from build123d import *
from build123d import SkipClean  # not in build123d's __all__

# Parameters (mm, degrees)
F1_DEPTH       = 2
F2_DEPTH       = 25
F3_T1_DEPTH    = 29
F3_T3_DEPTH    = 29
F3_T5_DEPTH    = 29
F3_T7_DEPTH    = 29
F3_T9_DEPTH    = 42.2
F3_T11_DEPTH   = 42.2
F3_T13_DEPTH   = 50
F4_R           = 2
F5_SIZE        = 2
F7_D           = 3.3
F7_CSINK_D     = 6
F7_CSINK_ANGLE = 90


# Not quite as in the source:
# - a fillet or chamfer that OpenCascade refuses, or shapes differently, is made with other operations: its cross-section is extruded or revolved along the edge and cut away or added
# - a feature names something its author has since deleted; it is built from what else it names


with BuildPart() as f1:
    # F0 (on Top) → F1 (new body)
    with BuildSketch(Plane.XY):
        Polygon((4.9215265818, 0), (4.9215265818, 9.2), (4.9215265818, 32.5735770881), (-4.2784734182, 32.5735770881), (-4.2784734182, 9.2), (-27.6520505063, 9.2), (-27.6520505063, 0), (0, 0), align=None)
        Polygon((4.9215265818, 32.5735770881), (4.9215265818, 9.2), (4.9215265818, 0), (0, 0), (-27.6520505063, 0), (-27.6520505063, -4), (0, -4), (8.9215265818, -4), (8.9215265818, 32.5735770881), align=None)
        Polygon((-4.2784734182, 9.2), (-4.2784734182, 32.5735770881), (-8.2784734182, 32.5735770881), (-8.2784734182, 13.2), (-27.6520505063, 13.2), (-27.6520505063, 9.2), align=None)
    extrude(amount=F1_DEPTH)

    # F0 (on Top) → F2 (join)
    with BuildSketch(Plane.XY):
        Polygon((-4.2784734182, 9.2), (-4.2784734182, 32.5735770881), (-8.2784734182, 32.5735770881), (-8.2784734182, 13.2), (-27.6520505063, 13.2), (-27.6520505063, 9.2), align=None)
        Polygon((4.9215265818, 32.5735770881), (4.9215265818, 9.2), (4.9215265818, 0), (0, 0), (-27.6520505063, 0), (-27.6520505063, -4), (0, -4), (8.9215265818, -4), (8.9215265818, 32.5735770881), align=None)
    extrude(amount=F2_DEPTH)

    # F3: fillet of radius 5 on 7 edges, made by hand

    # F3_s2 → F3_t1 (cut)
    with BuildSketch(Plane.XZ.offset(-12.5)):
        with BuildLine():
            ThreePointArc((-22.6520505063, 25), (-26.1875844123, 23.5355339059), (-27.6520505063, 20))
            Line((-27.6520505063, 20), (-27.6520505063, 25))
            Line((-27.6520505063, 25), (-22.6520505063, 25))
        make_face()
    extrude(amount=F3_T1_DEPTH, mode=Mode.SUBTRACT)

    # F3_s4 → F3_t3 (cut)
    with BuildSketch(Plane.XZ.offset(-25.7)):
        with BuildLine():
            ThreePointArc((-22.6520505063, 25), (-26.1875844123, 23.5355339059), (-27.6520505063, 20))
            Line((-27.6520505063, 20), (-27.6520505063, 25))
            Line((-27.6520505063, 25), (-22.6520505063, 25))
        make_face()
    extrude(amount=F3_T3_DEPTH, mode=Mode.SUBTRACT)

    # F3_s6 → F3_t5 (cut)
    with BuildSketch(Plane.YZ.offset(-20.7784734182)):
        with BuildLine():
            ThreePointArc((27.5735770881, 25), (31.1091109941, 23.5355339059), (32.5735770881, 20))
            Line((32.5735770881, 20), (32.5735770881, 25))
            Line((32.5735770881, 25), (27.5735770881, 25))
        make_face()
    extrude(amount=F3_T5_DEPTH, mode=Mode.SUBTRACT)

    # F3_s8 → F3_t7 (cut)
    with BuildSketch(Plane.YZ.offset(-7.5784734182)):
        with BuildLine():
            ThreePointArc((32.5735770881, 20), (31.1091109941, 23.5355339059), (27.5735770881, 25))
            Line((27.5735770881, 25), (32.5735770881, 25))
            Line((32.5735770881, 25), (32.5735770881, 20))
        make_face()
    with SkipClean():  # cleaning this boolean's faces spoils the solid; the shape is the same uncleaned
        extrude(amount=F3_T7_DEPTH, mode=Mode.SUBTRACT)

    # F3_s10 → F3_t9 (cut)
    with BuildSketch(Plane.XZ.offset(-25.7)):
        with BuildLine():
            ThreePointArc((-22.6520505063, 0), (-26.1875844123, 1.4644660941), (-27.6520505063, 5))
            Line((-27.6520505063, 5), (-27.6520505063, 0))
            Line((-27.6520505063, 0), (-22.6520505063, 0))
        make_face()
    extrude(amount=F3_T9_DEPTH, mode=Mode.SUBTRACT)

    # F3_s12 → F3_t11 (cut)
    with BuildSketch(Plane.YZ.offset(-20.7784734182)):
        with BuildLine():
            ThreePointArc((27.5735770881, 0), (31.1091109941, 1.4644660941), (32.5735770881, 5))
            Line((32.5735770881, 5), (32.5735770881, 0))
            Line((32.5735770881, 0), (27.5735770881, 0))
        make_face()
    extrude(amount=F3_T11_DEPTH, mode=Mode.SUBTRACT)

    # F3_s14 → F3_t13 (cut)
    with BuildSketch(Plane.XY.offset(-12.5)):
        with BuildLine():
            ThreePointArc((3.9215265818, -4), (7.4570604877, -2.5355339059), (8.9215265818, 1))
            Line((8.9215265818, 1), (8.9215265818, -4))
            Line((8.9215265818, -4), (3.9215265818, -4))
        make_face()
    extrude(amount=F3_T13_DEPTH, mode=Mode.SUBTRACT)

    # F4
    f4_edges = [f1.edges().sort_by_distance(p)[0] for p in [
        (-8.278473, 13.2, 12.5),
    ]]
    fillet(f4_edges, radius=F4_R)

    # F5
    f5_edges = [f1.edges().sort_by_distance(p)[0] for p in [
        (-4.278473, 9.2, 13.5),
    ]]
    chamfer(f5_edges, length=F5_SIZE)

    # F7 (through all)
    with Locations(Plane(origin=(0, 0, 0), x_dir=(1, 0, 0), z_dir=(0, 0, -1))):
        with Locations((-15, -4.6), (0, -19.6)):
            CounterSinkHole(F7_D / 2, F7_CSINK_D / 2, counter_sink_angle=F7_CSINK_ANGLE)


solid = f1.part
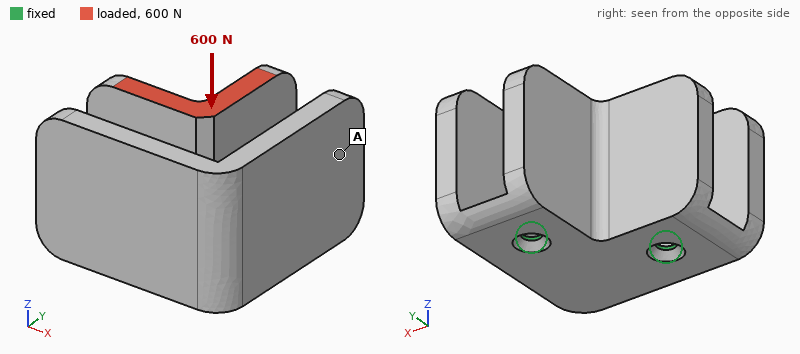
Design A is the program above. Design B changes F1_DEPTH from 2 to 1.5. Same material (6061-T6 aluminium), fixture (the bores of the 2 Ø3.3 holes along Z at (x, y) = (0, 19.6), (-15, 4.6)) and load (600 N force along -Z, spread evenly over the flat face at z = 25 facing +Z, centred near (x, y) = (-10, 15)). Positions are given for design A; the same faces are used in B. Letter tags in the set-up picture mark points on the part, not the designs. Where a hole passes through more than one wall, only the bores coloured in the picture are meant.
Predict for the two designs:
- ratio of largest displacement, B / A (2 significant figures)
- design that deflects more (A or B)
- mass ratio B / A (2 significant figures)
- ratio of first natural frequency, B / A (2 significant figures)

3.7
B
0.98
0.53
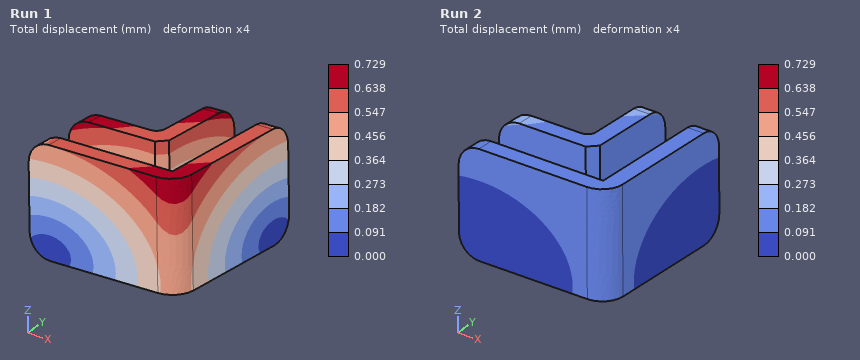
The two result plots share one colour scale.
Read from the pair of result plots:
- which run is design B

Run 1
